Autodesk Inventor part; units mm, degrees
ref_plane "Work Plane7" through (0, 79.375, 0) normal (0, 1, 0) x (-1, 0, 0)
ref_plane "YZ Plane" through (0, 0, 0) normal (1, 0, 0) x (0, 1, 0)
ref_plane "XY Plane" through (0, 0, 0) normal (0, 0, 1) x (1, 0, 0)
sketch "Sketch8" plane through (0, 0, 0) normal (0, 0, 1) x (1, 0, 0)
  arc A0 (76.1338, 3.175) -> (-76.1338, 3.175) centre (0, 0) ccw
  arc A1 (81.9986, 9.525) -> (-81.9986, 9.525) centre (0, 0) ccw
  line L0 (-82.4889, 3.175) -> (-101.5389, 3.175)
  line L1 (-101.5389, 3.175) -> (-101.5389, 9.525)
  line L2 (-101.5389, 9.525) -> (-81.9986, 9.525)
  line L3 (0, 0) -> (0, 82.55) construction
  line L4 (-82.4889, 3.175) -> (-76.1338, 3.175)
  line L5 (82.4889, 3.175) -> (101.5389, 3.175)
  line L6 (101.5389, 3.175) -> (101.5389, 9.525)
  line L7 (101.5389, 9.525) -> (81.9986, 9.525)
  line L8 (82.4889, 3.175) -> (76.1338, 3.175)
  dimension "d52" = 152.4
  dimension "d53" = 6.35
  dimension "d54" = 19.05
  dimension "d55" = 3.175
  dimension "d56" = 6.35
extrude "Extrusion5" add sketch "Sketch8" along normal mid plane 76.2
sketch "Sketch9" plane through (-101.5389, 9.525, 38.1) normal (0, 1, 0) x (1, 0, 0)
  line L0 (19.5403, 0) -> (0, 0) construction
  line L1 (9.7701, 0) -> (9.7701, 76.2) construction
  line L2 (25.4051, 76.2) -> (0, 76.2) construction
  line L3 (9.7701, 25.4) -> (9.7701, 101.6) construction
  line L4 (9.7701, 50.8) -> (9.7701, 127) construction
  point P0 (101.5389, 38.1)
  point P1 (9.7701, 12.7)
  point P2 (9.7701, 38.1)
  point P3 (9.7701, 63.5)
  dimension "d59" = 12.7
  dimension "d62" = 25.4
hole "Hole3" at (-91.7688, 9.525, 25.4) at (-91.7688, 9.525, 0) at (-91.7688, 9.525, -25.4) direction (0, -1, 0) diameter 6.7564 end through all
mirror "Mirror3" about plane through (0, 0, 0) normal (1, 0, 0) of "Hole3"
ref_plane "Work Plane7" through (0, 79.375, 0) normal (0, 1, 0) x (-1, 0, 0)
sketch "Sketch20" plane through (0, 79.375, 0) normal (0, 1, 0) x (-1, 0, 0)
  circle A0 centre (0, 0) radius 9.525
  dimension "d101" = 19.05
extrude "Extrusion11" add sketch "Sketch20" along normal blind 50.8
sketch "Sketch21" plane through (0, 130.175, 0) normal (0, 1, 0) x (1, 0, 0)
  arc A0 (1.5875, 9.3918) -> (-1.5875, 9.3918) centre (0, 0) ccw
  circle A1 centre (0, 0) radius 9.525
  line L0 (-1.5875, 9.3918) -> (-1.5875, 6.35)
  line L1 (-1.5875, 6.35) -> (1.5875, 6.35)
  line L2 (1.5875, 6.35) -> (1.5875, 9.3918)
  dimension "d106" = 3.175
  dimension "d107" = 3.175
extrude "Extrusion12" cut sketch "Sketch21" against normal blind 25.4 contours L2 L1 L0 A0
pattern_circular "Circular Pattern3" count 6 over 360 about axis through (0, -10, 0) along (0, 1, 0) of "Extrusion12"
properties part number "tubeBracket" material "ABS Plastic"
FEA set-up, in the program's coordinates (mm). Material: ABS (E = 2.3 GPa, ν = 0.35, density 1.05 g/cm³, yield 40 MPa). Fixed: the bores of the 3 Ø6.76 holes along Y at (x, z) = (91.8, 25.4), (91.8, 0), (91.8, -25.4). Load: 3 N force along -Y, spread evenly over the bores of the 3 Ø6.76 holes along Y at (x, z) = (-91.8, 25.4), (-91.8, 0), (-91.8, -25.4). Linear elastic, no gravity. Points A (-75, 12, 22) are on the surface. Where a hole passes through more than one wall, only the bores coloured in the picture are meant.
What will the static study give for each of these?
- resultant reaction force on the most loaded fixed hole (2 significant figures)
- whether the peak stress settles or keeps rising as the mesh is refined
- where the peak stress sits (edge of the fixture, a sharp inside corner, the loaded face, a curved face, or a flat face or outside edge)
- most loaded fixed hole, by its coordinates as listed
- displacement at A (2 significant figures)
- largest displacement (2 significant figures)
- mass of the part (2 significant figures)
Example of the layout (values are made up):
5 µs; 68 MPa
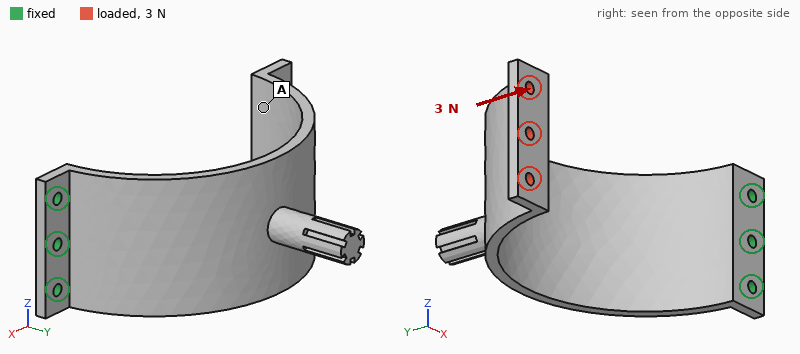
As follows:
4.8 N; keeps rising; edge of the fixture; (91.8, 0); 2.0 mm; 2.5 mm; 150 g
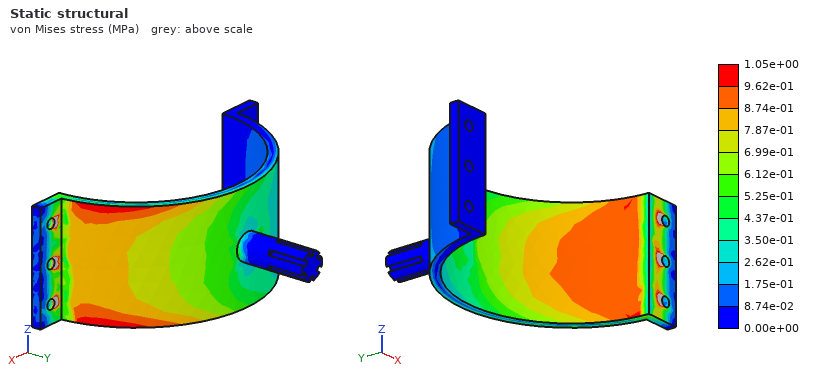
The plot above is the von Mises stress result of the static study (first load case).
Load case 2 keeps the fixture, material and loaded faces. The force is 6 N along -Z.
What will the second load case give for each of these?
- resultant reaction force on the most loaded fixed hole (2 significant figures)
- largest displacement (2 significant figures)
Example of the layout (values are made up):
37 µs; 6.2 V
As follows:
20 N; 2.3 mm
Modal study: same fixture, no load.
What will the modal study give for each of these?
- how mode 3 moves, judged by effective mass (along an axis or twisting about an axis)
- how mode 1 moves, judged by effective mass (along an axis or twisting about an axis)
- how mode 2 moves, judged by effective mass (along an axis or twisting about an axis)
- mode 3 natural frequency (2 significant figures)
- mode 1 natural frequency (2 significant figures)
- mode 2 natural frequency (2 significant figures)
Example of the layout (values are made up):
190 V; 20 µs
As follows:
along X; along Y; along Z; 84 Hz; 26 Hz; 46 Hz
